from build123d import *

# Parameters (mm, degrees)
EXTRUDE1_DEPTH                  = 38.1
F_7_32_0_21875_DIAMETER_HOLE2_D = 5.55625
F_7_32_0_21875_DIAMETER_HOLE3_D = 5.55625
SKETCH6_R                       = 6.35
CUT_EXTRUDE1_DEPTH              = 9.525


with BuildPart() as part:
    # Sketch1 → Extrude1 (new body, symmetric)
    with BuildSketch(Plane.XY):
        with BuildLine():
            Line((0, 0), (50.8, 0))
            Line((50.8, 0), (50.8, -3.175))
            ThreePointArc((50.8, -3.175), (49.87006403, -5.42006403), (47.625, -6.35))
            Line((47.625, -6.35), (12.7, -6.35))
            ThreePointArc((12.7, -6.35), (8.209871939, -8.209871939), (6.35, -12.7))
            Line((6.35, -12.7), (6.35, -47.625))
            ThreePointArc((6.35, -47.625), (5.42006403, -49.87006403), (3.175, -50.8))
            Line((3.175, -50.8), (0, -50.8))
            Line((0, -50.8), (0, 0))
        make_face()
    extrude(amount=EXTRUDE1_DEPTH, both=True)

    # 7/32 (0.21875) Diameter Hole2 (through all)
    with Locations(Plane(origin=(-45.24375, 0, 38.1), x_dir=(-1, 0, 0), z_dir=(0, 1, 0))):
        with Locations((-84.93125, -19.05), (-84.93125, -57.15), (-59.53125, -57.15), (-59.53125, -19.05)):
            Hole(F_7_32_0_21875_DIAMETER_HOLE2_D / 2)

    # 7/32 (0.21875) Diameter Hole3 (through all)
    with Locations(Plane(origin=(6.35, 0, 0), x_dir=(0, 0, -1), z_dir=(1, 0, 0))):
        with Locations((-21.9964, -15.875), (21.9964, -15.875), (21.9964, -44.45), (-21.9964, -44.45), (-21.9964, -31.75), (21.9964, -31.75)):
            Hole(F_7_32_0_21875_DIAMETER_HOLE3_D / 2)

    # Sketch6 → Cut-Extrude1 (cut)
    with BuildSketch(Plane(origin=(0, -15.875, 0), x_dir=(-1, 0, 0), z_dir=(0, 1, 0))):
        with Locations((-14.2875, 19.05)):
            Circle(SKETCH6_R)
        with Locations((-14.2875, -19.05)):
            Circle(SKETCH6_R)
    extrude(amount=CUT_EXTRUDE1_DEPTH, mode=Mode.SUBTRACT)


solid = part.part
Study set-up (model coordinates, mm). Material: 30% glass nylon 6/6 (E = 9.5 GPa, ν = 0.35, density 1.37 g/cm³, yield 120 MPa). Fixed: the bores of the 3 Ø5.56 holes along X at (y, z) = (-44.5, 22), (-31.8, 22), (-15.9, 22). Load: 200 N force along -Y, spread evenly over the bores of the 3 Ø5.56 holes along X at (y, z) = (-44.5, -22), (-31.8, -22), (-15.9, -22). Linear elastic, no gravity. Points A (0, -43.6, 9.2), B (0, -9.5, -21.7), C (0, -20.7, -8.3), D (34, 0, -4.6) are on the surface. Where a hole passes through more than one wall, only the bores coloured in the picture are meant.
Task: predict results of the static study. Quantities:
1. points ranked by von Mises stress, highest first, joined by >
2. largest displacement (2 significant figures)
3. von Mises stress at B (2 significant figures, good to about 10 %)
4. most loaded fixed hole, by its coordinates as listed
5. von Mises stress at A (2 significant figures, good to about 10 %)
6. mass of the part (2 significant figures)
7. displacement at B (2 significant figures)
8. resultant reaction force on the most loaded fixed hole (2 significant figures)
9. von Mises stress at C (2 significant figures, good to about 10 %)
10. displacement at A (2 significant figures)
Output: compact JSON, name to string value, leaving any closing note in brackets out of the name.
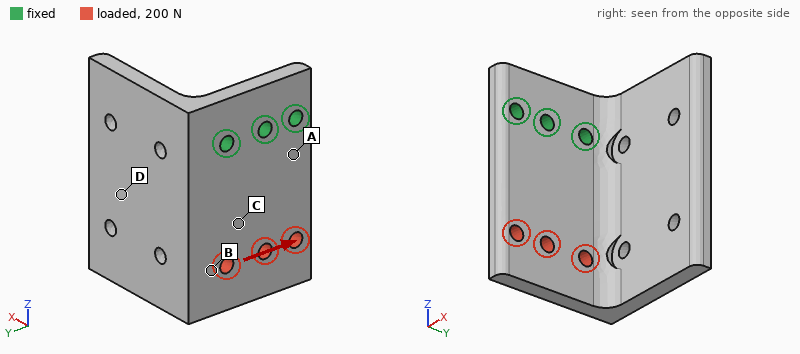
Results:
{"points ranked by von Mises stress, highest first, joined by >": "A > C > B > D", "largest displacement": "30 µm", "von Mises stress at B": "0.95 MPa", "most loaded fixed hole, by its coordinates as listed": "(-15.9, 22)", "von Mises stress at A": "2.1 MPa", "mass of the part": "61 g", "displacement at B": "22 µm", "resultant reaction force on the most loaded fixed hole": "300 N", "von Mises stress at C": "1.5 MPa", "displacement at A": "5.0 µm"}
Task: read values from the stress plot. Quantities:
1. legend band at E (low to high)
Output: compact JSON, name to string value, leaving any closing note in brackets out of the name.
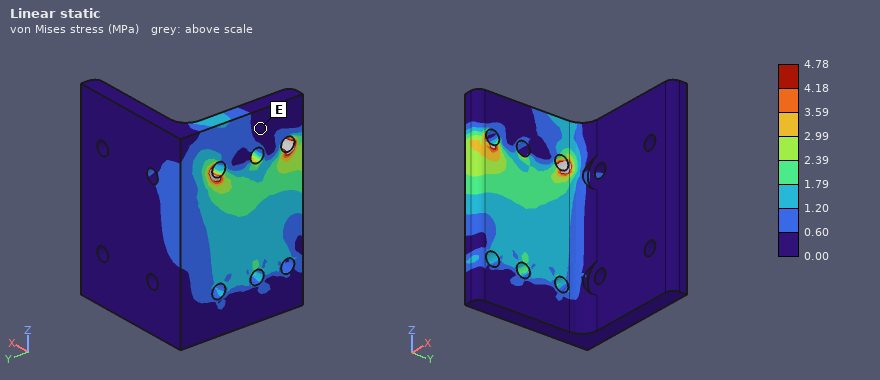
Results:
{"legend band at E": "0.00 to 0.60 MPa"}
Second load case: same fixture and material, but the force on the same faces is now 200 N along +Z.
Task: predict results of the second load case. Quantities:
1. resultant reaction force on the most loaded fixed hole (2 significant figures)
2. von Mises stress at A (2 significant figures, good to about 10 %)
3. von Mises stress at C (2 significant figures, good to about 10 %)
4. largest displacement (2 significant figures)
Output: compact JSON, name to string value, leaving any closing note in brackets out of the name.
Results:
{"resultant reaction force on the most loaded fixed hole": "73 N", "von Mises stress at A": "0.91 MPa", "von Mises stress at C": "0.64 MPa", "largest displacement": "5.1 µm"}
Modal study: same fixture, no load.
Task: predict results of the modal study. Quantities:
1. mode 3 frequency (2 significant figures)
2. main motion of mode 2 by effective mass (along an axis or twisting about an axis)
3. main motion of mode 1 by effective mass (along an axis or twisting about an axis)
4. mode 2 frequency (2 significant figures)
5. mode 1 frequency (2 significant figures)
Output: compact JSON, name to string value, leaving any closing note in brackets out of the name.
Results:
{"mode 3 frequency": "1700 Hz", "main motion of mode 2 by effective mass": "along Y", "main motion of mode 1 by effective mass": "along X", "mode 2 frequency": "840 Hz", "mode 1 frequency": "640 Hz"}
